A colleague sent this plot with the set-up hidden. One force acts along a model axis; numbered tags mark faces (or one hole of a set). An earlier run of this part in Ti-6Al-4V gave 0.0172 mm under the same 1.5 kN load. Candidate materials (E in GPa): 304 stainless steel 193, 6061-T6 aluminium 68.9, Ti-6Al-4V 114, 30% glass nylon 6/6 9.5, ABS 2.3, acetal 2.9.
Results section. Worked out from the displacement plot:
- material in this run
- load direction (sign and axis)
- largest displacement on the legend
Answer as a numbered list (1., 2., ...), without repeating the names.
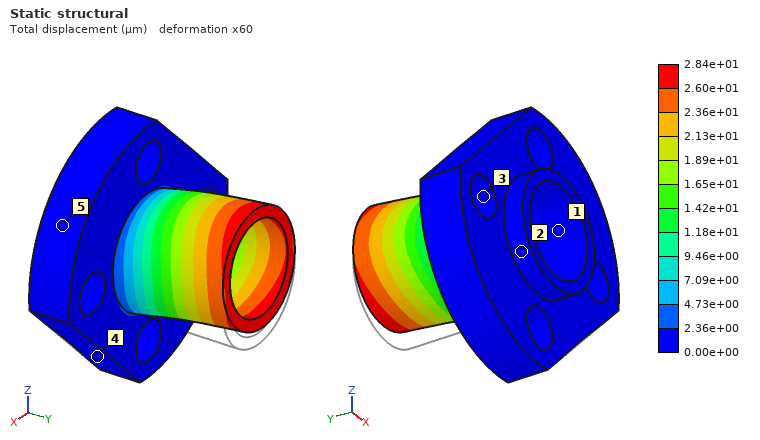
1. 6061-T6 aluminium
2. +Z
3. 2.84e+01 µm
